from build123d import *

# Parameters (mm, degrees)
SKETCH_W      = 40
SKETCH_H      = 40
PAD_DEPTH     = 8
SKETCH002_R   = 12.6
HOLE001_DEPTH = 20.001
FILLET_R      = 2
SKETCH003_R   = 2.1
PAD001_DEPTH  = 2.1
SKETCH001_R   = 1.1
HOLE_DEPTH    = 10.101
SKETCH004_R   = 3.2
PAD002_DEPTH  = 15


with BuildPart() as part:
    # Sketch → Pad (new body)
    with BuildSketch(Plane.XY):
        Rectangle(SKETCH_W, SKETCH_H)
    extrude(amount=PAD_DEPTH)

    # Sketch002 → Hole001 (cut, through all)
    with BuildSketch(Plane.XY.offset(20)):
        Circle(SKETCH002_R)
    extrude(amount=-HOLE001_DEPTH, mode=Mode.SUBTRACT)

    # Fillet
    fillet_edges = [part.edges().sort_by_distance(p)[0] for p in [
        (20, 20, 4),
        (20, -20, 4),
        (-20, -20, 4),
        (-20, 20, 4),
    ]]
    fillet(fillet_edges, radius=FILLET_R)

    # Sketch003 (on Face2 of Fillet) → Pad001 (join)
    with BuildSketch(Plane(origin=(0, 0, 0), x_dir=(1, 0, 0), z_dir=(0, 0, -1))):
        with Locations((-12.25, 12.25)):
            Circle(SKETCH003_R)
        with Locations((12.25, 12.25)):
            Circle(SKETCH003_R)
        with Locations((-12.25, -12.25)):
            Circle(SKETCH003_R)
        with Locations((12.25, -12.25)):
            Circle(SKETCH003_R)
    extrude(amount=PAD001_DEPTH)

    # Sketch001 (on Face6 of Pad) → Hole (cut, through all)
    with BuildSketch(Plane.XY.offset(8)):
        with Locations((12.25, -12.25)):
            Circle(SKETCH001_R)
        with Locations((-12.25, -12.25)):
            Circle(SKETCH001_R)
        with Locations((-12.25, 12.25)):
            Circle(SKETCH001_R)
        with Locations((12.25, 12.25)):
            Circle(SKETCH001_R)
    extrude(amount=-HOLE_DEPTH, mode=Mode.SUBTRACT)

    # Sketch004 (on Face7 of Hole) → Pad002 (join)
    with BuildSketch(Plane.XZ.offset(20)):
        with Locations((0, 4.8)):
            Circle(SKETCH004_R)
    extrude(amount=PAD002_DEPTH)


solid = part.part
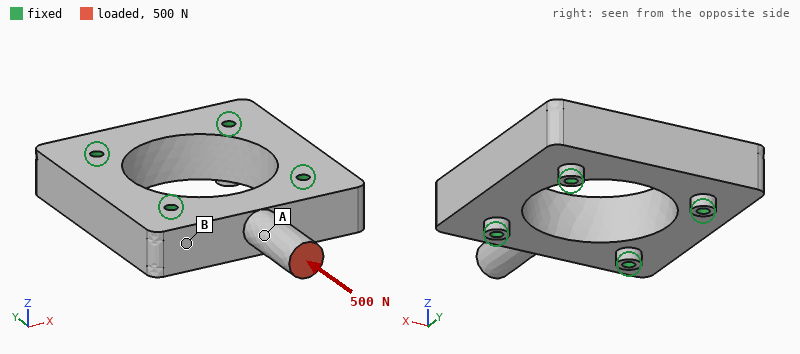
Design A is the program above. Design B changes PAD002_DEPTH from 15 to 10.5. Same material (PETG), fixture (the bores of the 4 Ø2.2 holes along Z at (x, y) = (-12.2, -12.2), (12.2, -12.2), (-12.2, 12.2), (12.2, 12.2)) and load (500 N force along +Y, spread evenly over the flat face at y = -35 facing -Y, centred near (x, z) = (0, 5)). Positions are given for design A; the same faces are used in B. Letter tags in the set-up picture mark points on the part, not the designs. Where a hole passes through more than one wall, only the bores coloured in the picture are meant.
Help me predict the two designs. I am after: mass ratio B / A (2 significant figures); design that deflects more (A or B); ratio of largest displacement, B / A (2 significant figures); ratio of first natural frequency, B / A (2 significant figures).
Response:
0.98
A
0.83
1.6
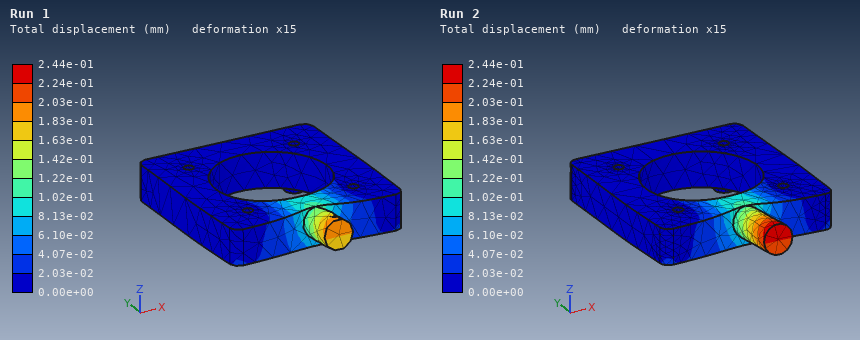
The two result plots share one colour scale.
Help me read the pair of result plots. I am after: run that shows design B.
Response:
Run 1
